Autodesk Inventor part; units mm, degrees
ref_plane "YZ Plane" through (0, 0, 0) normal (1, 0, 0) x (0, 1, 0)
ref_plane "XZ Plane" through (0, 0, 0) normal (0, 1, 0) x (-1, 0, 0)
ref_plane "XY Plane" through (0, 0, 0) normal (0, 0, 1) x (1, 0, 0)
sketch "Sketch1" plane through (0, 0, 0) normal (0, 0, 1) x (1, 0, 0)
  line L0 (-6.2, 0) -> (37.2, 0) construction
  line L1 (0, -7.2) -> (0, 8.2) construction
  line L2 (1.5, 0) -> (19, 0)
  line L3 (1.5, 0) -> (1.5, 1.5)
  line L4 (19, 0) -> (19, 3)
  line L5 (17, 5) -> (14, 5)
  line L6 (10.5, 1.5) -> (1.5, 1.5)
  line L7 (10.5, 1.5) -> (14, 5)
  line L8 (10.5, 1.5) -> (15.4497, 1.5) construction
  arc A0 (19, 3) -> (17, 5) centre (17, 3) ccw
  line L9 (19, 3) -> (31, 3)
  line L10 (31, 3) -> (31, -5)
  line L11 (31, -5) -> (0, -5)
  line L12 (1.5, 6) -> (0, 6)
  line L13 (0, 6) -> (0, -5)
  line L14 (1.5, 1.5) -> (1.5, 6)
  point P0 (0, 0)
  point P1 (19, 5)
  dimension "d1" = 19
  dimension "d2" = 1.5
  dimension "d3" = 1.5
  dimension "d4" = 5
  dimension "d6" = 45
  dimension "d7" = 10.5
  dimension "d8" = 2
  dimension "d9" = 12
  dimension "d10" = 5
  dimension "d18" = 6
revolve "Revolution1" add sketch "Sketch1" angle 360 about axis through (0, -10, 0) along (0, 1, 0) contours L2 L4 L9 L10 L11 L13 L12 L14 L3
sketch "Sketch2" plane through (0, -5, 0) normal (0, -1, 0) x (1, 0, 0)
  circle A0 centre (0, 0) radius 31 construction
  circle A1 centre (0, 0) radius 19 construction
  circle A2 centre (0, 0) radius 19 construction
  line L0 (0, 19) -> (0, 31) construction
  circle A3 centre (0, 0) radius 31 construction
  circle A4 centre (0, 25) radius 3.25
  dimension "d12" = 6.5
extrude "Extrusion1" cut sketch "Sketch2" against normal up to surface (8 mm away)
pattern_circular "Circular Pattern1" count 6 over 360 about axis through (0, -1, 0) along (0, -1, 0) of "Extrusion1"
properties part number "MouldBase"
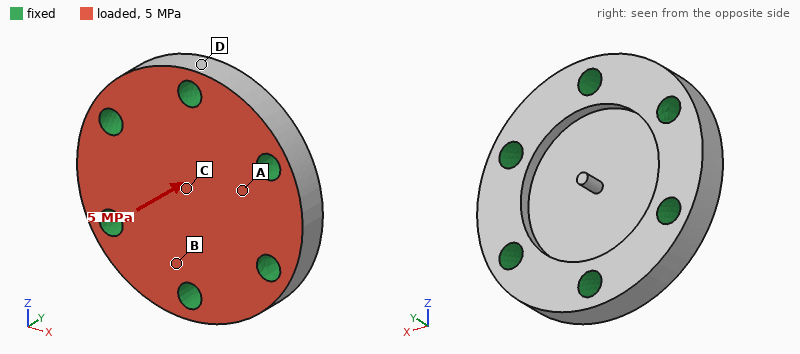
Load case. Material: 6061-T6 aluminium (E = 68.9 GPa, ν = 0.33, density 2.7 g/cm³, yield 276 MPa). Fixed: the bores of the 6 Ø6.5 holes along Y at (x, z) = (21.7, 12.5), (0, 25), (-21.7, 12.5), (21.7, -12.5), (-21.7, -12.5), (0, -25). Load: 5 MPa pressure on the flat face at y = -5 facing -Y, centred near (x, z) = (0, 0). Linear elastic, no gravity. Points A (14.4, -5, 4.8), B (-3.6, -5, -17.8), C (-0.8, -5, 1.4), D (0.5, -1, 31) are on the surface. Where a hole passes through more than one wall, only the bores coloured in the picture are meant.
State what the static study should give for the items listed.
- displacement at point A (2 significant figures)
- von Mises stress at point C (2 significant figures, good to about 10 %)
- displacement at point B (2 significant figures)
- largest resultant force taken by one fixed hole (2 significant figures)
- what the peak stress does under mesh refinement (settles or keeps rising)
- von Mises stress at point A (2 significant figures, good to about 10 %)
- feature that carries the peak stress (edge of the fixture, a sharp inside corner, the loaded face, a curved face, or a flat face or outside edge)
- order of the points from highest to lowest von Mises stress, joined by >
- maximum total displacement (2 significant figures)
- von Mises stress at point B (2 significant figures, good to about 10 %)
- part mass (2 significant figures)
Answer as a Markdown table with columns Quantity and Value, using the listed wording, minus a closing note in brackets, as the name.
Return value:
| Quantity | Value |
|---|---|
| displacement at point A | 11 µm |
| von Mises stress at point C | 46 MPa |
| displacement at point B | 6.2 µm |
| largest resultant force taken by one fixed hole | 2.4 kN |
| what the peak stress does under mesh refinement | keeps rising |
| von Mises stress at point A | 19 MPa |
| feature that carries the peak stress | edge of the fixture |
| order of the points from highest to lowest von Mises stress, joined by > | C > B > A > D |
| maximum total displacement | 28 µm |
| von Mises stress at point B | 31 MPa |
| part mass | 52 g |
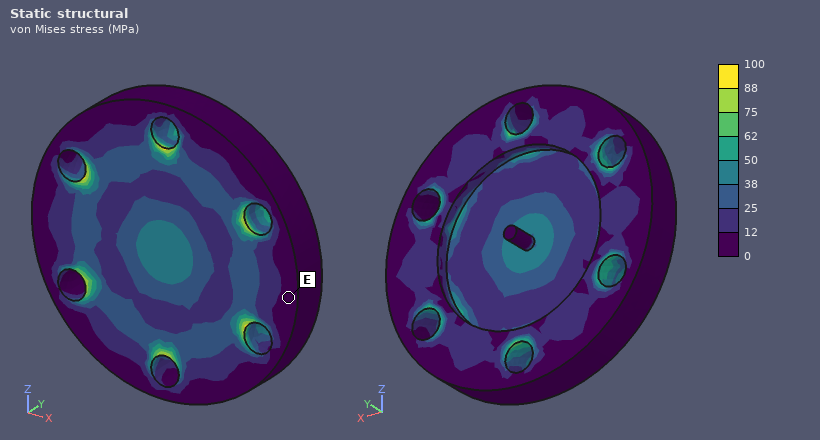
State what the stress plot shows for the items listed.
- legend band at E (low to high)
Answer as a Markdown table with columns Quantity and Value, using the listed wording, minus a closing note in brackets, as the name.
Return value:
| Quantity | Value |
|---|---|
| legend band at E | 0 to 12 MPa |
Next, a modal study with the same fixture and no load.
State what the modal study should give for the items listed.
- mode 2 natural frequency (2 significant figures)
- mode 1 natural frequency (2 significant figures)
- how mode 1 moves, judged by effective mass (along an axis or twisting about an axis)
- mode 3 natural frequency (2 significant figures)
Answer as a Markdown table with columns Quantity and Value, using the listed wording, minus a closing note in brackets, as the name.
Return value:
| Quantity | Value |
|---|---|
| mode 2 natural frequency | 39 kHz |
| mode 1 natural frequency | 22 kHz |
| how mode 1 moves, judged by effective mass | along Y |
| mode 3 natural frequency | 39 kHz |
